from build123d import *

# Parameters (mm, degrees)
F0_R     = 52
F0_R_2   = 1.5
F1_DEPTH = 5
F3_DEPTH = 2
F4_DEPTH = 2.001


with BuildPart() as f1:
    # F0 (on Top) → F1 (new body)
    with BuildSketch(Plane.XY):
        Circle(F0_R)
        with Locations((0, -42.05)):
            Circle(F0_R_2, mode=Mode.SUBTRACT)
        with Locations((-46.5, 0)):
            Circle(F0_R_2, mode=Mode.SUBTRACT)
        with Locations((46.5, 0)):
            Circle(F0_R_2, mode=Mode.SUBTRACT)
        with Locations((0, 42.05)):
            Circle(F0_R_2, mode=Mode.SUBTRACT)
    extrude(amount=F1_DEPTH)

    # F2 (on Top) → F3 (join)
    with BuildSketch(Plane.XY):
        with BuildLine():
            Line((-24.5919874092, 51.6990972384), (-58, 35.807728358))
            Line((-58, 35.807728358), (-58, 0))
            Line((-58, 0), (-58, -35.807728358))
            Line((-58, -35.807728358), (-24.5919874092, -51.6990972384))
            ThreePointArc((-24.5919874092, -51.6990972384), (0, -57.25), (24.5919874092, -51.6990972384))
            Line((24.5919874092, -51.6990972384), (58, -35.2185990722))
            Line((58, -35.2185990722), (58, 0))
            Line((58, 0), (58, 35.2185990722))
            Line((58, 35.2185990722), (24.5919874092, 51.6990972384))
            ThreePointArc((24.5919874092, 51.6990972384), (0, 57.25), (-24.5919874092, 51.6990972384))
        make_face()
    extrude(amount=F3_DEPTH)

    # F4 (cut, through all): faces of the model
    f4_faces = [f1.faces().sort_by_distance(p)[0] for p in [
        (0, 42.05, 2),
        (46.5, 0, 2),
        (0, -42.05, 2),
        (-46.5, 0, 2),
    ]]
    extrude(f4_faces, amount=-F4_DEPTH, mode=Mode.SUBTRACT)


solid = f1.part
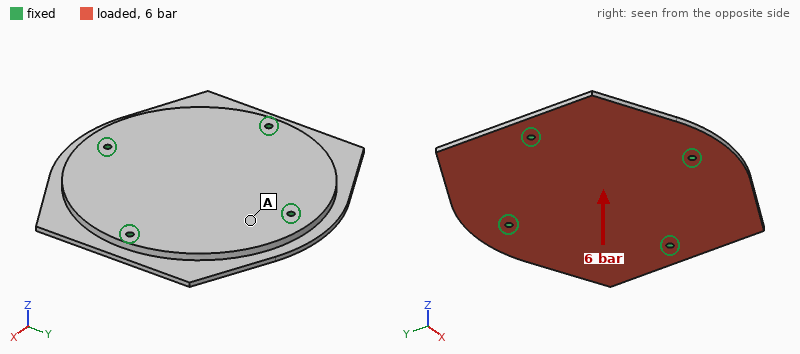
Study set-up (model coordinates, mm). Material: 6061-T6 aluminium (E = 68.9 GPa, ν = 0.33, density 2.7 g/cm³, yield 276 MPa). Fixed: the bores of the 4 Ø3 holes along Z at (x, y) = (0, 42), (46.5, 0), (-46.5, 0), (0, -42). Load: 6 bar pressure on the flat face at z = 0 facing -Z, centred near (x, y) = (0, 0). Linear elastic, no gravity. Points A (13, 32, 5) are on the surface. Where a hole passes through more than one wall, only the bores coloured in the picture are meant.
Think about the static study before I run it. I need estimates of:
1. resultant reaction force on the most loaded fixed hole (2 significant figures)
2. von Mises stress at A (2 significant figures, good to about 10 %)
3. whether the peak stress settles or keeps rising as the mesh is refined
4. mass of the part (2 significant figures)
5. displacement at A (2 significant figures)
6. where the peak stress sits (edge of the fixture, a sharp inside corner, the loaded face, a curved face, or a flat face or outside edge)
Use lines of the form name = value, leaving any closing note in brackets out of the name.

resultant reaction force on the most loaded fixed hole = 1.7 kN
von Mises stress at A = 33 MPa
whether the peak stress settles or keeps rising as the mesh is refined = keeps rising
mass of the part = 130 g
displacement at A = 0.043 mm
where the peak stress sits = edge of the fixture
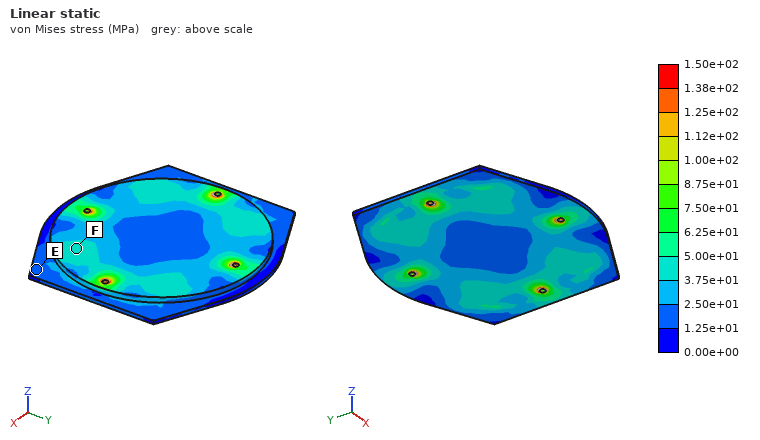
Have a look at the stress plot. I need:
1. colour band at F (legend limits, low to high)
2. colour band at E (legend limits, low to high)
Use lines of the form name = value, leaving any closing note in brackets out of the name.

colour band at F = 3.75e+01 to 5.00e+01 MPa
colour band at E = 1.25e+01 to 2.50e+01 MPa
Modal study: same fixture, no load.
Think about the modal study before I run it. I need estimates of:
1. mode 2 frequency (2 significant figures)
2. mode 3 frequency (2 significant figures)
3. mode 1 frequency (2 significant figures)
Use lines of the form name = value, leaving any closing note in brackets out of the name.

mode 2 frequency = 3900 Hz
mode 3 frequency = 3900 Hz
mode 1 frequency = 3500 Hz
